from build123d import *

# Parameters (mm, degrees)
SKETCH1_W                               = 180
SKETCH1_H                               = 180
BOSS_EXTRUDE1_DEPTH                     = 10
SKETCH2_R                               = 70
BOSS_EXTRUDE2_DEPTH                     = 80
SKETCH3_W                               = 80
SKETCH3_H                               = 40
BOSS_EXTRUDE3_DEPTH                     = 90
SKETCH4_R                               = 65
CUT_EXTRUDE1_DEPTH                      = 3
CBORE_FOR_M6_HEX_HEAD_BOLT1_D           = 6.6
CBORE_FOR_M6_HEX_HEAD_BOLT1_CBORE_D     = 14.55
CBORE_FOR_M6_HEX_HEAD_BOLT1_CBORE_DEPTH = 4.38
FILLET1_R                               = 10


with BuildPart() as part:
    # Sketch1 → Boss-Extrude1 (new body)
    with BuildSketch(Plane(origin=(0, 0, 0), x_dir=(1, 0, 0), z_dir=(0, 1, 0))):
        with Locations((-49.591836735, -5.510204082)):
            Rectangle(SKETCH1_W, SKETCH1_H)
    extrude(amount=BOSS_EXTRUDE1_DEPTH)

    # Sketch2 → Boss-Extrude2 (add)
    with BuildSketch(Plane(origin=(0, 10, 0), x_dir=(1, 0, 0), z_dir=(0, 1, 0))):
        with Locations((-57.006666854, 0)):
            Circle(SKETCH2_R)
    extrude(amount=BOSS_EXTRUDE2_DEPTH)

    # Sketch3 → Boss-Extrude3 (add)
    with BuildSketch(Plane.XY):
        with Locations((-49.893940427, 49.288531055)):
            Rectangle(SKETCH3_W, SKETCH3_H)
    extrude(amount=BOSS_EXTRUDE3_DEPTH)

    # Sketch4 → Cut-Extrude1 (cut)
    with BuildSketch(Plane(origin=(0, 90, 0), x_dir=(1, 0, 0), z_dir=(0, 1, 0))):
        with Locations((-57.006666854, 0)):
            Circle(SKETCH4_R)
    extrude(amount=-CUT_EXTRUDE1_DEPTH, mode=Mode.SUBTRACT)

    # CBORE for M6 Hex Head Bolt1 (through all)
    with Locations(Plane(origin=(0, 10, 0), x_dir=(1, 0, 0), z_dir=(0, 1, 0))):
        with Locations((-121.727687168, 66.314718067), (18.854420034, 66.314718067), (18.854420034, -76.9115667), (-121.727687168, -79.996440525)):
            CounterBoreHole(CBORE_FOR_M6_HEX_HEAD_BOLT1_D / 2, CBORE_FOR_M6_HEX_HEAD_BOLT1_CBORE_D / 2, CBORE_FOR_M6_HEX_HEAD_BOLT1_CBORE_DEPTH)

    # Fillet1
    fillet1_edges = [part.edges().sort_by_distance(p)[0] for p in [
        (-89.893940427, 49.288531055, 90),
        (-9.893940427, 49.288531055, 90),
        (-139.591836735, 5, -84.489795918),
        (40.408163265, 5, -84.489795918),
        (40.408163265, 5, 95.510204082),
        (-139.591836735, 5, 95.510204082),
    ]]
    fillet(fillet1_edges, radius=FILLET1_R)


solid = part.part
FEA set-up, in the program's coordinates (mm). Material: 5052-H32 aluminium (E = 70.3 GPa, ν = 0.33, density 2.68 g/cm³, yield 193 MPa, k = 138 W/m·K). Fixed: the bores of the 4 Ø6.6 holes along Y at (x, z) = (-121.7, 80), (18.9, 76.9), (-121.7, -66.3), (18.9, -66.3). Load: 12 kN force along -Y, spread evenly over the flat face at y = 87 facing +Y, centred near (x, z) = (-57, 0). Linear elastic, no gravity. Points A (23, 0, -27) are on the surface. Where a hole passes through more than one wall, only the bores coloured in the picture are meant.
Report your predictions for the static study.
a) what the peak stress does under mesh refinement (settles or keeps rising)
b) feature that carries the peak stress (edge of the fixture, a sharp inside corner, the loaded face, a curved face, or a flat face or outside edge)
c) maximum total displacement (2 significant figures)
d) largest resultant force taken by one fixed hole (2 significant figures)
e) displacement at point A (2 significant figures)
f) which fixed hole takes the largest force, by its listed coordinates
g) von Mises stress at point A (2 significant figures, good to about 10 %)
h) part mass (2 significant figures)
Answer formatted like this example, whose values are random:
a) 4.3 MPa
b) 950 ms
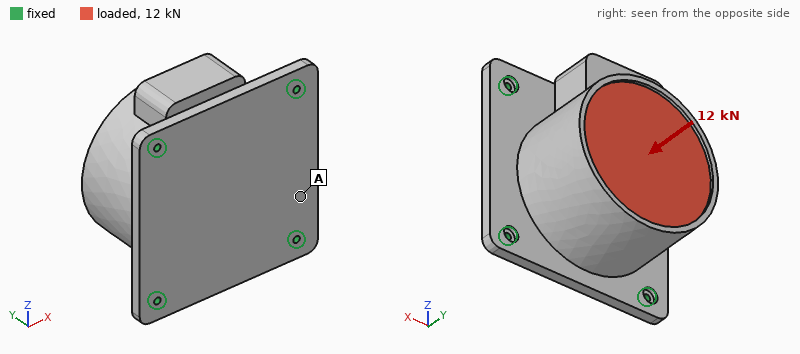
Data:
a) keeps rising
b) edge of the fixture
c) 100 µm
d) 5.1 kN
e) 67 µm
f) (-121.7, -66.3)
g) 18 MPa
h) 4.3 kg
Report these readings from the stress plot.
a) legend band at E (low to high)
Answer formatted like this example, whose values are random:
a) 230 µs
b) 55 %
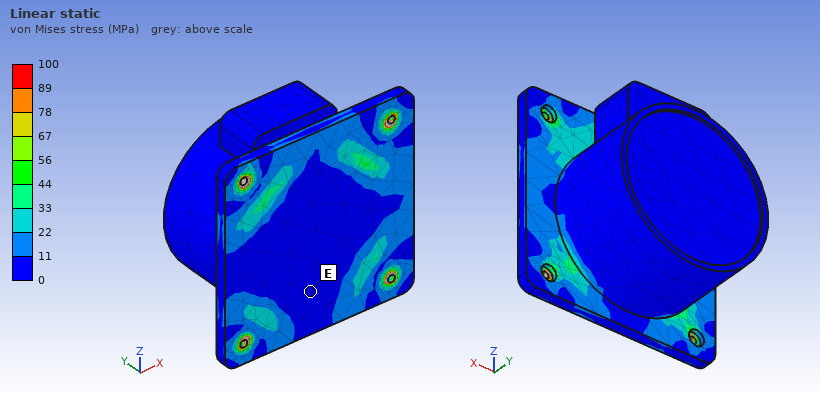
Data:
a) 0 to 11 MPa
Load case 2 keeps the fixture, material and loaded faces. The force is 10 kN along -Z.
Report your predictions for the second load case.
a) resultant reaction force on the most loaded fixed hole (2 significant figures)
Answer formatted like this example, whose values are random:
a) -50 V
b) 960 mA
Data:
a) 5.7 kN
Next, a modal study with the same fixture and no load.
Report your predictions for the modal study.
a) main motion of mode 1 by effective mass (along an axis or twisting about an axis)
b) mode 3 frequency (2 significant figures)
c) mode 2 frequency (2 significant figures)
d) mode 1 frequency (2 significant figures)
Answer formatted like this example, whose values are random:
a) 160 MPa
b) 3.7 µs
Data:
a) along Y
b) 1200 Hz
c) 1100 Hz
d) 910 Hz
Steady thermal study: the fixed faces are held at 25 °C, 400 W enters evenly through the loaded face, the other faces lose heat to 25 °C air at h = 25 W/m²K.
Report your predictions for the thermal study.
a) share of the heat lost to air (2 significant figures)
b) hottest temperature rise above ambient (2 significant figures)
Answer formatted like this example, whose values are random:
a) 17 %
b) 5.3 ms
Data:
a) 28 %
b) 64 K
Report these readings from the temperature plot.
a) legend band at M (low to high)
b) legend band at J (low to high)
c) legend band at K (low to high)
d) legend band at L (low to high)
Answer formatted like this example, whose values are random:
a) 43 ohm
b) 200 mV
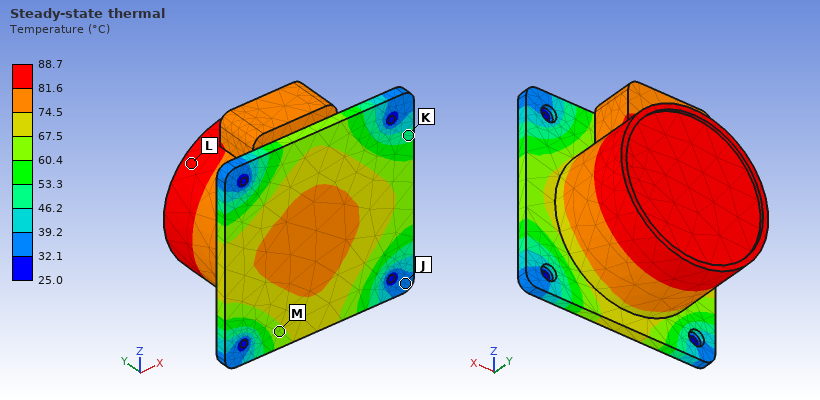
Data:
a) 60.4 to 67.5 °C
b) 32.1 to 39.2 °C
c) 46.2 to 53.3 °C
d) 81.6 to 88.7 °C
